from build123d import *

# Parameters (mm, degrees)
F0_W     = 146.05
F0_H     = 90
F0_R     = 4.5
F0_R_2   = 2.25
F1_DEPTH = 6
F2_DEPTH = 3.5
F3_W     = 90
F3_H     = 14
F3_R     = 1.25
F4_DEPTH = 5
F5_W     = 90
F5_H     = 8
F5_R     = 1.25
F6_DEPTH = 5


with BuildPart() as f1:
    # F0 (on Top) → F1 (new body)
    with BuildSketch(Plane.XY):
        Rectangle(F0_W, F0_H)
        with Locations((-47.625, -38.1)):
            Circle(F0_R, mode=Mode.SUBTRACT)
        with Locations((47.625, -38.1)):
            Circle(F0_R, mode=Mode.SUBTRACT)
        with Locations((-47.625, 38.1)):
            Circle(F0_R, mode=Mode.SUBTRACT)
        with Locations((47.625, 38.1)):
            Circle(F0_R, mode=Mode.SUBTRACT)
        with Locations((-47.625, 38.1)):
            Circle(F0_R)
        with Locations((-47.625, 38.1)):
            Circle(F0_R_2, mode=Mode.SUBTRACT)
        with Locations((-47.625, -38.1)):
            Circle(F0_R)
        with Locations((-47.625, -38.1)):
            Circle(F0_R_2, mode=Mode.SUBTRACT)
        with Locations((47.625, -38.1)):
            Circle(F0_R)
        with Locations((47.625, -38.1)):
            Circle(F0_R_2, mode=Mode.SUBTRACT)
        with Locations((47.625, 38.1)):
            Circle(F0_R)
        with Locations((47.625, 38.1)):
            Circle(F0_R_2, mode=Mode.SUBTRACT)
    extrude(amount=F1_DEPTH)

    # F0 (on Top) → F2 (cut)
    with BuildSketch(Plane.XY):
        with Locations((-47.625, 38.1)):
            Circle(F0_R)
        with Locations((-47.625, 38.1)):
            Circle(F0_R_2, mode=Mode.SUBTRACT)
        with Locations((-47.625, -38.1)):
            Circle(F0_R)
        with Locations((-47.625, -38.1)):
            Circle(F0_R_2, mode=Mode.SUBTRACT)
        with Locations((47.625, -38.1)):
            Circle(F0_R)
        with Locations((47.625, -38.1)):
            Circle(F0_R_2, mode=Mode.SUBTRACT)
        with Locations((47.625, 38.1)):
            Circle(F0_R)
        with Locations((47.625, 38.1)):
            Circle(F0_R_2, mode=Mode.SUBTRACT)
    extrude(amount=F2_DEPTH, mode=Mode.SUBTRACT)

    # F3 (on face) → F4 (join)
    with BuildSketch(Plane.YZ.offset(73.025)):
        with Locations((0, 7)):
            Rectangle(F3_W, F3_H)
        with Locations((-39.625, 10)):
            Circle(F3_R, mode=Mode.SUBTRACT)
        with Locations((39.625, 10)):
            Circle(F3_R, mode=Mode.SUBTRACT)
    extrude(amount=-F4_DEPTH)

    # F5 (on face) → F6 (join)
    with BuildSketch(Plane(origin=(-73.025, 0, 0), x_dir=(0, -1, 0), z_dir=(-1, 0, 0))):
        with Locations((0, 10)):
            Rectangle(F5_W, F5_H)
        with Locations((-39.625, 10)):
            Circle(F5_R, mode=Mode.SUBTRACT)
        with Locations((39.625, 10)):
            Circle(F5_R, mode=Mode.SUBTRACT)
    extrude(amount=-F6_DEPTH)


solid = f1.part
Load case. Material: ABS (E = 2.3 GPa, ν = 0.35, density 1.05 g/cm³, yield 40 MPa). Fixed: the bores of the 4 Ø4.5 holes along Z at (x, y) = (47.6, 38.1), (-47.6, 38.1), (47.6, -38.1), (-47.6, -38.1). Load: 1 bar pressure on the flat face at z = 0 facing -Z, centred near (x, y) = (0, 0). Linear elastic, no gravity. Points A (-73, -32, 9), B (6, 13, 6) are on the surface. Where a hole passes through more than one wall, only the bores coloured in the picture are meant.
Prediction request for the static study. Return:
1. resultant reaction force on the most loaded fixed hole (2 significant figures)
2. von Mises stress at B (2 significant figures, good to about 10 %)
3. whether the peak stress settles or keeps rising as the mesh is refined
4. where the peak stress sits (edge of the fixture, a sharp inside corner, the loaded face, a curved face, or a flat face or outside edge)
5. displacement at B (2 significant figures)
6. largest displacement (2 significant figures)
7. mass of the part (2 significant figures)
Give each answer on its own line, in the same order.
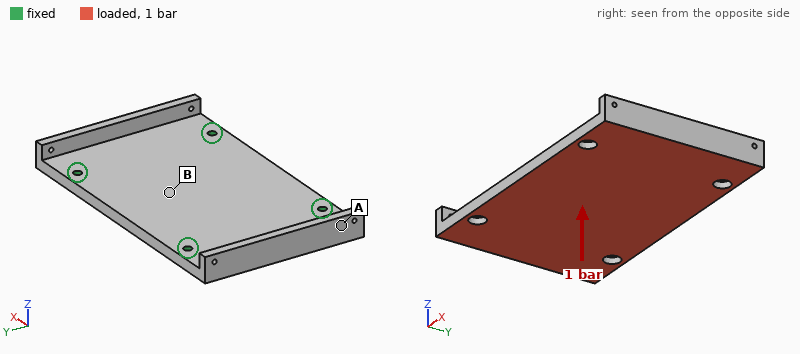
470 N
7.0 MPa
keeps rising
edge of the fixture
1.2 mm
1.2 mm
89 g
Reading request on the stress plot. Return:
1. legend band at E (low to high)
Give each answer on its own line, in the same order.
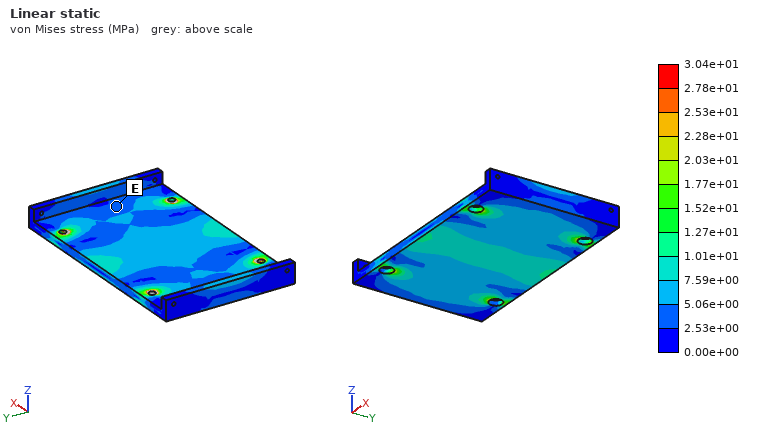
2.53e+00 to 5.06e+00 MPa
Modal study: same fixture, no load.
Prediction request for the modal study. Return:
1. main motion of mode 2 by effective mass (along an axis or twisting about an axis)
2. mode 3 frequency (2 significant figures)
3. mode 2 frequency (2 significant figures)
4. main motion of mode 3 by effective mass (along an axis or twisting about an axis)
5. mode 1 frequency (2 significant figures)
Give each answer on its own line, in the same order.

twisting about Y
840 Hz
810 Hz
along Z
580 Hz
